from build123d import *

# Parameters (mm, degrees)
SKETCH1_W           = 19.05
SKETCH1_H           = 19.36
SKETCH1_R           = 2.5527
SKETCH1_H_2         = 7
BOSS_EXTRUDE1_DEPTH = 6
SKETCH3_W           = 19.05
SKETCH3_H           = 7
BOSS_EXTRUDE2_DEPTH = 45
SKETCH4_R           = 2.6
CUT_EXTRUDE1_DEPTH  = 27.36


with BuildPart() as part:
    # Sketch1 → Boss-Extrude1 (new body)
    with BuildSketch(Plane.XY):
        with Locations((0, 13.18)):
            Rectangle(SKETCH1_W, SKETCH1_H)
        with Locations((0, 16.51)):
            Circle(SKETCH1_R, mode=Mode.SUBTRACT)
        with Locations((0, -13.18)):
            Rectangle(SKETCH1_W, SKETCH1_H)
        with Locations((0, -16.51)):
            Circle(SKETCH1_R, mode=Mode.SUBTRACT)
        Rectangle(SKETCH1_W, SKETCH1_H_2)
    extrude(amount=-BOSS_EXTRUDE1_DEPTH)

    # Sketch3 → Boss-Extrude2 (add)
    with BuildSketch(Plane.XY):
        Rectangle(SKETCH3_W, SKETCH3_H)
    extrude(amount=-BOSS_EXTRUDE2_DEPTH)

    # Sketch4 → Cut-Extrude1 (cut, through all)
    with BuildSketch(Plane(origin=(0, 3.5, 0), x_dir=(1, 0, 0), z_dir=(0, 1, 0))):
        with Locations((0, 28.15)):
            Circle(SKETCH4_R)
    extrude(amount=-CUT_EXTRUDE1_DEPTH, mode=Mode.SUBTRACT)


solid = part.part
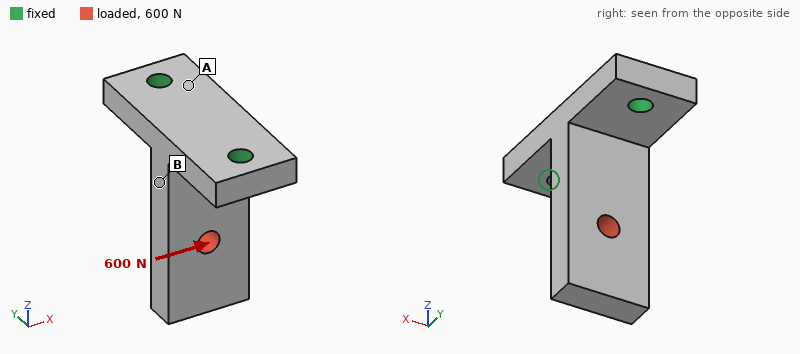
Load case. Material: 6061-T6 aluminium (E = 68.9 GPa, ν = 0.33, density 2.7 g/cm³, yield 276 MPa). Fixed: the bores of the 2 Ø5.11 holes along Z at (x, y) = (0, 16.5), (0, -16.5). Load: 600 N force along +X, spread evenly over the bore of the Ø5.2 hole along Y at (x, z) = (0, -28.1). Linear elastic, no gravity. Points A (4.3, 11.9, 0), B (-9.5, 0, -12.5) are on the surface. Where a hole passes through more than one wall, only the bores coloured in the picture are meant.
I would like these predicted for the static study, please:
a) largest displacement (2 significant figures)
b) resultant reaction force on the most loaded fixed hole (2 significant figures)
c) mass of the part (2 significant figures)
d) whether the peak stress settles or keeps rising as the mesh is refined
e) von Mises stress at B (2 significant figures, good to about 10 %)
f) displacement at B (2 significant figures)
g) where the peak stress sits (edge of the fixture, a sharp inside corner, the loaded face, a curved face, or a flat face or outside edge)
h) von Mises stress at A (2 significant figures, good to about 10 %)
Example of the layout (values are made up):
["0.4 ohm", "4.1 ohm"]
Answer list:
["0.15 mm", "300 N", "27 g", "keeps rising", "23 MPa", "0.044 mm", "edge of the fixture", "44 MPa"]
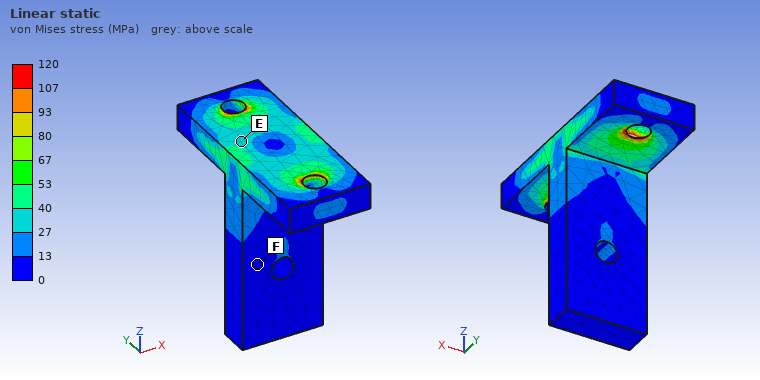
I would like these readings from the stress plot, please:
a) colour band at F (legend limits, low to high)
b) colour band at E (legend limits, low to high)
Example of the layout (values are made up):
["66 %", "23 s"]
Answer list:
["0 to 13 MPa", "27 to 40 MPa"]
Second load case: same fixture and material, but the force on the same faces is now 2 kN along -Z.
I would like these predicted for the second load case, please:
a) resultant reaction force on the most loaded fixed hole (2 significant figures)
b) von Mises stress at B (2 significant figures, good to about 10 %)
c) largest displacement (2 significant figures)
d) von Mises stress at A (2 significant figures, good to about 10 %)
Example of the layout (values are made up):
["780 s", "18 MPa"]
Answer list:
["1.0 kN", "14 MPa", "23 µm", "23 MPa"]
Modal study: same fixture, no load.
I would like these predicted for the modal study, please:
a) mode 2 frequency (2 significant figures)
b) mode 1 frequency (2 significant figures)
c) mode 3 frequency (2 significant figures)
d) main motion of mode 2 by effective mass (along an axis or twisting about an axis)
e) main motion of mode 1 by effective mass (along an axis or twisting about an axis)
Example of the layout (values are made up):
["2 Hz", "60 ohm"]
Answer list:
["3500 Hz", "3100 Hz", "12 kHz", "along X", "along Y"]
